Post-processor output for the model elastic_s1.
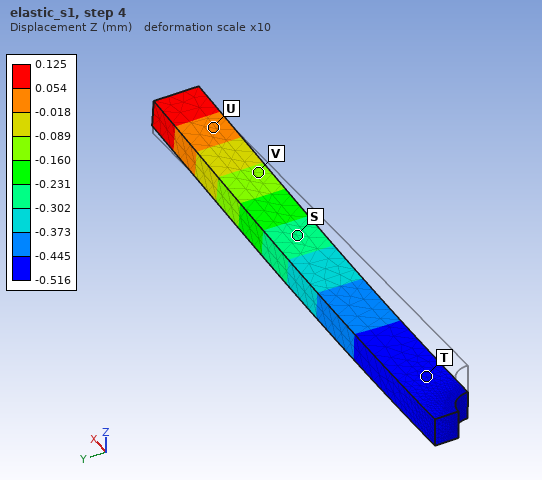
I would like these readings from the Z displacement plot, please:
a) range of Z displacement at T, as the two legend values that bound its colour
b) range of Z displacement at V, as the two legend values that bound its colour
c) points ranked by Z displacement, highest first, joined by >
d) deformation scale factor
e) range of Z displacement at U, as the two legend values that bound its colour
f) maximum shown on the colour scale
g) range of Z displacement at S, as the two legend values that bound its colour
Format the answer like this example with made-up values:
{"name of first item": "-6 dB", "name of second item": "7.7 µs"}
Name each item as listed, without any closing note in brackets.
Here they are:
{"range of Z displacement at T, as the two legend values that bound its colour": "-0.516 to -0.445 mm", "range of Z displacement at V, as the two legend values that bound its colour": "-0.160 to -0.089 mm", "points ranked by Z displacement, highest first, joined by >": "U > V > S > T", "deformation scale factor": "10", "range of Z displacement at U, as the two legend values that bound its colour": "-0.018 to 0.054 mm", "maximum shown on the colour scale": "0.125 mm", "range of Z displacement at S, as the two legend values that bound its colour": "-0.302 to -0.231 mm"}
